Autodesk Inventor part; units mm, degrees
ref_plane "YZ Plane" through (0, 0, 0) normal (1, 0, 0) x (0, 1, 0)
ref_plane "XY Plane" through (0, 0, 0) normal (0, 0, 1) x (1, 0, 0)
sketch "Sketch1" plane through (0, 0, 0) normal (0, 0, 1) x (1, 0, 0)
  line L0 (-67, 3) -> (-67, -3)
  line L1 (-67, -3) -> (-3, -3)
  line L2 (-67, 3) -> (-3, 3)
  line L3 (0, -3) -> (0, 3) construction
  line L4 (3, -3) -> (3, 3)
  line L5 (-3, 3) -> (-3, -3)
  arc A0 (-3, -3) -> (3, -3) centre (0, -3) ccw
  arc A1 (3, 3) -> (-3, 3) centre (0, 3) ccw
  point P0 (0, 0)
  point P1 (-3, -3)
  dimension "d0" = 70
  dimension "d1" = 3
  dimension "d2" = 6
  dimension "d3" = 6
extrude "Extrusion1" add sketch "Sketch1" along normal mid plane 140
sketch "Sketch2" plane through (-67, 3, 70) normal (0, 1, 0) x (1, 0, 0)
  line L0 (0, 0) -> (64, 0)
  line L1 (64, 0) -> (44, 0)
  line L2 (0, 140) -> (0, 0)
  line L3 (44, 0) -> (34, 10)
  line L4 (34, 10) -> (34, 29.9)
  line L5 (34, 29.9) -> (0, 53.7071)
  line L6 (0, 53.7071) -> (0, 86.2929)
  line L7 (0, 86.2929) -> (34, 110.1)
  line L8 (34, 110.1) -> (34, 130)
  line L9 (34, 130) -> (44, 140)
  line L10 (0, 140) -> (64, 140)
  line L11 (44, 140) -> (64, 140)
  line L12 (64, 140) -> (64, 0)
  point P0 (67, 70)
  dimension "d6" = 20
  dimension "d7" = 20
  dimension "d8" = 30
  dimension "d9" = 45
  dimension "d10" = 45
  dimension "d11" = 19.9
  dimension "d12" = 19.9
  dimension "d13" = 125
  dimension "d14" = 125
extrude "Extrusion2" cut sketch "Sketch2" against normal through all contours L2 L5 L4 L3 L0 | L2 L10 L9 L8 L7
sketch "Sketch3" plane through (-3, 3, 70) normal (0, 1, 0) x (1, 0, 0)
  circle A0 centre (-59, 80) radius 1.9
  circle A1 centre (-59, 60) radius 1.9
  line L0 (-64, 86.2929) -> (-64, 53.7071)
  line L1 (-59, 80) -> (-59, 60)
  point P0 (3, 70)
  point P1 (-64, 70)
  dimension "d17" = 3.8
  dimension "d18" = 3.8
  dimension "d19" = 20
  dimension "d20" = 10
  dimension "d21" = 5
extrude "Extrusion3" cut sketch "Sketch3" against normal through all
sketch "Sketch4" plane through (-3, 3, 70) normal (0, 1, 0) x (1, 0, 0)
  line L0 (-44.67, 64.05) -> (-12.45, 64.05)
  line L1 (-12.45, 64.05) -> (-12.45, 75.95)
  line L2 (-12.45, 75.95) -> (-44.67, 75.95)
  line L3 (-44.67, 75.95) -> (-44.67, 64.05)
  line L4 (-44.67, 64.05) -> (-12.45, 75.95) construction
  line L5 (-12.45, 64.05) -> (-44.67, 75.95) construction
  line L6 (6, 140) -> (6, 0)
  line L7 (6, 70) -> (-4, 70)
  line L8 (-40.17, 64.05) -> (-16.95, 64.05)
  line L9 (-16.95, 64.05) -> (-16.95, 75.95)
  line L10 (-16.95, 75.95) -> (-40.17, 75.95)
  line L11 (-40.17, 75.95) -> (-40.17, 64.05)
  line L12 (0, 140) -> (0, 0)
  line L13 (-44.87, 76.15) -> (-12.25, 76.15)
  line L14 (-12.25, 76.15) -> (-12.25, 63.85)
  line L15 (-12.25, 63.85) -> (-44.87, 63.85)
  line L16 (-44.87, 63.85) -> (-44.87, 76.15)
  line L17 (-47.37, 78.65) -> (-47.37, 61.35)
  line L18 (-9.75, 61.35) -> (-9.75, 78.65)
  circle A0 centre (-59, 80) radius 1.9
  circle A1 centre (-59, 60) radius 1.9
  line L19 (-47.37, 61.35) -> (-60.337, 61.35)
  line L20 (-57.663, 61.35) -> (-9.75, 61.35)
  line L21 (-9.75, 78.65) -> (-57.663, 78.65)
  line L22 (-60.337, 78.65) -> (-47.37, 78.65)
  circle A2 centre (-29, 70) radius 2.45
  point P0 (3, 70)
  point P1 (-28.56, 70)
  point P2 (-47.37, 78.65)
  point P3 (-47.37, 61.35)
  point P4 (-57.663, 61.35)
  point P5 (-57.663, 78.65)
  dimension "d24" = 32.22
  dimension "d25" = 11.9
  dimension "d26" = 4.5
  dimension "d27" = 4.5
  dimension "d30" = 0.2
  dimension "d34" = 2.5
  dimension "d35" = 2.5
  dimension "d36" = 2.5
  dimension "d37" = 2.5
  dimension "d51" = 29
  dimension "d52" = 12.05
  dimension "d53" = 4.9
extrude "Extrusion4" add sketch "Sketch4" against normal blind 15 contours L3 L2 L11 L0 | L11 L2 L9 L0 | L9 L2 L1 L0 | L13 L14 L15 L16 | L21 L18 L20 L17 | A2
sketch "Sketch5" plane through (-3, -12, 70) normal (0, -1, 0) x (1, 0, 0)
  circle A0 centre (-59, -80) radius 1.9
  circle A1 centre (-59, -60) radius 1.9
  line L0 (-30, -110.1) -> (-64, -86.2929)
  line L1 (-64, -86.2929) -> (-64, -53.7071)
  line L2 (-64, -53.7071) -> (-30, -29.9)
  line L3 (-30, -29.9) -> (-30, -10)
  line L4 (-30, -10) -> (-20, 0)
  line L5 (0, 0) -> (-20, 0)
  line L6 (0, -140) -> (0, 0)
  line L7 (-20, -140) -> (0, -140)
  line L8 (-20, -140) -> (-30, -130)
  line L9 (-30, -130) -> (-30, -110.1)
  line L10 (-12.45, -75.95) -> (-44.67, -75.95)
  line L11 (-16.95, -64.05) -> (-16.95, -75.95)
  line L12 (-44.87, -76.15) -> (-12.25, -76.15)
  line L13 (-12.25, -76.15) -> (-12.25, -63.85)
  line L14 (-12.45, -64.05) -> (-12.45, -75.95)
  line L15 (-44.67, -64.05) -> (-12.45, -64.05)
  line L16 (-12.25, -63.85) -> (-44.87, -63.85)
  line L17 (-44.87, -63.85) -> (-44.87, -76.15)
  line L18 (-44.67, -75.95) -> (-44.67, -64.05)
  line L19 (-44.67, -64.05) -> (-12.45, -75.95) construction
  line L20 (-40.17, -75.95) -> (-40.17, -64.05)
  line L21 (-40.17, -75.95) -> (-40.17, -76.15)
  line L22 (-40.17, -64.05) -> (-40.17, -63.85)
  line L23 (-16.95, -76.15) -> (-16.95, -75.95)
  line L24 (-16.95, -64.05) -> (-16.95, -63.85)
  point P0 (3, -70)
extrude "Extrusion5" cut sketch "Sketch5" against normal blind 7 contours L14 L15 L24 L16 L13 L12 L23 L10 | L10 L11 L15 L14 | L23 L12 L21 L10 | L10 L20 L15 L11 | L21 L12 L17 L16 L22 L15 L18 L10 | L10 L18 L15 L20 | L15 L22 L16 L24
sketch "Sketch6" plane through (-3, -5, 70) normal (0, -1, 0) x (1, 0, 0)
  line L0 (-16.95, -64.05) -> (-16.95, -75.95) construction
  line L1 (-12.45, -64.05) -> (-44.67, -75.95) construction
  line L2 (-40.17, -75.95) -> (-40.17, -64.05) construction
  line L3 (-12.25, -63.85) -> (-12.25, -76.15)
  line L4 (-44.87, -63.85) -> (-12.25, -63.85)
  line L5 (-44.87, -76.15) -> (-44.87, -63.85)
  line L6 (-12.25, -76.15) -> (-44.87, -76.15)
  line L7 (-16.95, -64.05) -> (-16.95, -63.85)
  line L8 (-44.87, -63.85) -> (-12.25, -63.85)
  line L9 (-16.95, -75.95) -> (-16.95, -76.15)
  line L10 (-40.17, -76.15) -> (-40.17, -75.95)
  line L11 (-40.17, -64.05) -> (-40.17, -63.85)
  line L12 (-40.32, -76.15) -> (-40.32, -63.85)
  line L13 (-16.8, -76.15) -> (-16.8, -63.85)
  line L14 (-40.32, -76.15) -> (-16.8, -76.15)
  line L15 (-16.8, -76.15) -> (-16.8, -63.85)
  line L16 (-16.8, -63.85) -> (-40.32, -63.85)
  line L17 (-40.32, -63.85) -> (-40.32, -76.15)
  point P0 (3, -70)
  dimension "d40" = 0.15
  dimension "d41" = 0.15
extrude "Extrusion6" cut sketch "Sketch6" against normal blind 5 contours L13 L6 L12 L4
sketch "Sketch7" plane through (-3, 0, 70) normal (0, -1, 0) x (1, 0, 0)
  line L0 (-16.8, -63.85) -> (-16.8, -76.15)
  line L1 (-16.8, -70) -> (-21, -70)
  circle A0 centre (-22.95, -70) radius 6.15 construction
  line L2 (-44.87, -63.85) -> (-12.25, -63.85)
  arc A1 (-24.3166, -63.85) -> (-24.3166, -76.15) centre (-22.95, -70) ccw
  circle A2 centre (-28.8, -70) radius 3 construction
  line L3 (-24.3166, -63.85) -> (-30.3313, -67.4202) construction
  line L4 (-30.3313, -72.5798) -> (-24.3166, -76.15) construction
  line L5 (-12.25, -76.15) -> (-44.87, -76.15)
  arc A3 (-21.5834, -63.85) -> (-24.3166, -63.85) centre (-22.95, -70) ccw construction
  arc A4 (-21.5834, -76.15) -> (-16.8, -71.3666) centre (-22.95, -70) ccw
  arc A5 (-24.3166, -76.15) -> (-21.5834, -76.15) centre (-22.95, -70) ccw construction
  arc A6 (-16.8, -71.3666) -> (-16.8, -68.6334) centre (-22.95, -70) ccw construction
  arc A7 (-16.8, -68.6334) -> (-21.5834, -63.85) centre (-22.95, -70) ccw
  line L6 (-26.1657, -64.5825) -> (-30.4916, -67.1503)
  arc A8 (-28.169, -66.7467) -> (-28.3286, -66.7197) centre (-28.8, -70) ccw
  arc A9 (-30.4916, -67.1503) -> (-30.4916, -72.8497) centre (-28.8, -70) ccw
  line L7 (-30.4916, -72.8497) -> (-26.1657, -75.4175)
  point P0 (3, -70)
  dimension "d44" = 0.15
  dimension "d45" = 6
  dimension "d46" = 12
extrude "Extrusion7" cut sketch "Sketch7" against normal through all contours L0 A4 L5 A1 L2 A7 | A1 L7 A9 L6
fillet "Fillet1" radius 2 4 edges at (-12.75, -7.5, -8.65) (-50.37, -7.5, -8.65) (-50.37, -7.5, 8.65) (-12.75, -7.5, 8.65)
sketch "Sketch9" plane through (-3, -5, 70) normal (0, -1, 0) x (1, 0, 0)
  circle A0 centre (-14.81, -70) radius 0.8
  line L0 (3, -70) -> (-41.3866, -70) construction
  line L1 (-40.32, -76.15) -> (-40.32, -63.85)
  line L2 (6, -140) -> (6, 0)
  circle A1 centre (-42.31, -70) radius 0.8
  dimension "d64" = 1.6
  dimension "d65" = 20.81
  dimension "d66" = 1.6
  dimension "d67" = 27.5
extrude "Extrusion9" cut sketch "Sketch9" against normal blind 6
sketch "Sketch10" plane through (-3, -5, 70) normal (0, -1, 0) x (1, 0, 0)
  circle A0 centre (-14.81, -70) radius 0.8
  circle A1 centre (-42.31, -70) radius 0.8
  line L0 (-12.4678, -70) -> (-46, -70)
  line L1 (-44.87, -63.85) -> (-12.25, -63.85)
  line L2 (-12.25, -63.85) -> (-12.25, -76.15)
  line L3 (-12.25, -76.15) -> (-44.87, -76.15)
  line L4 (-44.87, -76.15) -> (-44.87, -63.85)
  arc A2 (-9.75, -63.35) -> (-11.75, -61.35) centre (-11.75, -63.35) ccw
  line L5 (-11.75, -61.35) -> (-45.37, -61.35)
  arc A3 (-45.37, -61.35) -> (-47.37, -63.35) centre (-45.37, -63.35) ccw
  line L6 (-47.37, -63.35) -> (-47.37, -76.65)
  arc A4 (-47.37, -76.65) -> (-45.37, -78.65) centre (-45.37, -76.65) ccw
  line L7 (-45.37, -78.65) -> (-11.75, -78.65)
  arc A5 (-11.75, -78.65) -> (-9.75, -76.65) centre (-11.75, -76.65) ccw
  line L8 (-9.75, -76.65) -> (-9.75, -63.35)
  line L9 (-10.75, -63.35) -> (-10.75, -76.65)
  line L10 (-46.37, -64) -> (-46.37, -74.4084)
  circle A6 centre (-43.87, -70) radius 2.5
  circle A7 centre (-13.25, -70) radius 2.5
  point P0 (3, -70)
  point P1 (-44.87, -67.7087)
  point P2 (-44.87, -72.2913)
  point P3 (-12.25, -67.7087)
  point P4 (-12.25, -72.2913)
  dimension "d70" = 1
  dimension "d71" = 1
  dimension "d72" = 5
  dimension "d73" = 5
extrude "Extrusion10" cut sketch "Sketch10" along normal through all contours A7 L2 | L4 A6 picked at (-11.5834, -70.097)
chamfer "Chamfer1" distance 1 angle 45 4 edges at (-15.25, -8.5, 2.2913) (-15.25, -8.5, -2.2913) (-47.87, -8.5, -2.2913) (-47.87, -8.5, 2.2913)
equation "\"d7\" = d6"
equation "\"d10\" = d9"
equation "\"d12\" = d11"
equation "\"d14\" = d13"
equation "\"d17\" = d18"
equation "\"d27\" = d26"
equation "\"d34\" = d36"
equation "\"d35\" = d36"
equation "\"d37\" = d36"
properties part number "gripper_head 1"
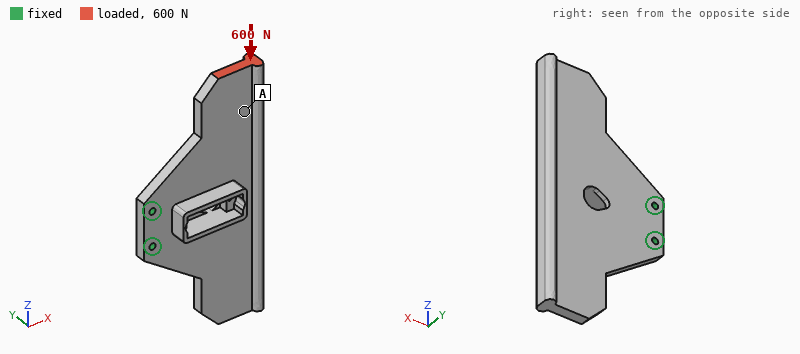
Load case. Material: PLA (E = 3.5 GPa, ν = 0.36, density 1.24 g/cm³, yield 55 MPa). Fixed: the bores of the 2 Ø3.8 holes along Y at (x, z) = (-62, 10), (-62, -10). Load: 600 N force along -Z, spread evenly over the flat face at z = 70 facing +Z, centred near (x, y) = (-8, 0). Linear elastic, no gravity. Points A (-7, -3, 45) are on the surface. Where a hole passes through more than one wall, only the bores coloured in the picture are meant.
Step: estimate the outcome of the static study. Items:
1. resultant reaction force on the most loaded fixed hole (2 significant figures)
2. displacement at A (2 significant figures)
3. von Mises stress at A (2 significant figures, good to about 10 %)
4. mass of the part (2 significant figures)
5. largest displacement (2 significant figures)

1.4 kN
0.73 mm
3.1 MPa
57 g
1.0 mm
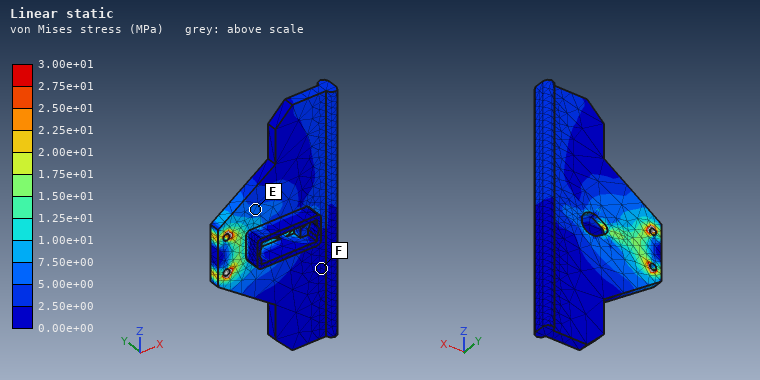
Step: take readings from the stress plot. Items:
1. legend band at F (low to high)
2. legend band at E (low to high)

0.00e+00 to 2.50e+00 MPa
5.00e+00 to 7.50e+00 MPa
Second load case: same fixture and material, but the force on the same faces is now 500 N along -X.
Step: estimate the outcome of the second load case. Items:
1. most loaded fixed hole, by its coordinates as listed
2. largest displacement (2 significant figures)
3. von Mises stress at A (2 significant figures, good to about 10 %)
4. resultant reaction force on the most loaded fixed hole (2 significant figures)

(-62, 10)
1.3 mm
4.4 MPa
1.8 kN
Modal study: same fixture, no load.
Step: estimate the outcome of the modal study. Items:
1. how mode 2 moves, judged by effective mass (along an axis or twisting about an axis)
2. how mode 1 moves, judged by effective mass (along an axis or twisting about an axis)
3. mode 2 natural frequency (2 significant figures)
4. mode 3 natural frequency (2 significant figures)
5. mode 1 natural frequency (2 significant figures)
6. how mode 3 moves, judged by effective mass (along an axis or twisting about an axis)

twisting about X
along Y
240 Hz
690 Hz
210 Hz
along Z
